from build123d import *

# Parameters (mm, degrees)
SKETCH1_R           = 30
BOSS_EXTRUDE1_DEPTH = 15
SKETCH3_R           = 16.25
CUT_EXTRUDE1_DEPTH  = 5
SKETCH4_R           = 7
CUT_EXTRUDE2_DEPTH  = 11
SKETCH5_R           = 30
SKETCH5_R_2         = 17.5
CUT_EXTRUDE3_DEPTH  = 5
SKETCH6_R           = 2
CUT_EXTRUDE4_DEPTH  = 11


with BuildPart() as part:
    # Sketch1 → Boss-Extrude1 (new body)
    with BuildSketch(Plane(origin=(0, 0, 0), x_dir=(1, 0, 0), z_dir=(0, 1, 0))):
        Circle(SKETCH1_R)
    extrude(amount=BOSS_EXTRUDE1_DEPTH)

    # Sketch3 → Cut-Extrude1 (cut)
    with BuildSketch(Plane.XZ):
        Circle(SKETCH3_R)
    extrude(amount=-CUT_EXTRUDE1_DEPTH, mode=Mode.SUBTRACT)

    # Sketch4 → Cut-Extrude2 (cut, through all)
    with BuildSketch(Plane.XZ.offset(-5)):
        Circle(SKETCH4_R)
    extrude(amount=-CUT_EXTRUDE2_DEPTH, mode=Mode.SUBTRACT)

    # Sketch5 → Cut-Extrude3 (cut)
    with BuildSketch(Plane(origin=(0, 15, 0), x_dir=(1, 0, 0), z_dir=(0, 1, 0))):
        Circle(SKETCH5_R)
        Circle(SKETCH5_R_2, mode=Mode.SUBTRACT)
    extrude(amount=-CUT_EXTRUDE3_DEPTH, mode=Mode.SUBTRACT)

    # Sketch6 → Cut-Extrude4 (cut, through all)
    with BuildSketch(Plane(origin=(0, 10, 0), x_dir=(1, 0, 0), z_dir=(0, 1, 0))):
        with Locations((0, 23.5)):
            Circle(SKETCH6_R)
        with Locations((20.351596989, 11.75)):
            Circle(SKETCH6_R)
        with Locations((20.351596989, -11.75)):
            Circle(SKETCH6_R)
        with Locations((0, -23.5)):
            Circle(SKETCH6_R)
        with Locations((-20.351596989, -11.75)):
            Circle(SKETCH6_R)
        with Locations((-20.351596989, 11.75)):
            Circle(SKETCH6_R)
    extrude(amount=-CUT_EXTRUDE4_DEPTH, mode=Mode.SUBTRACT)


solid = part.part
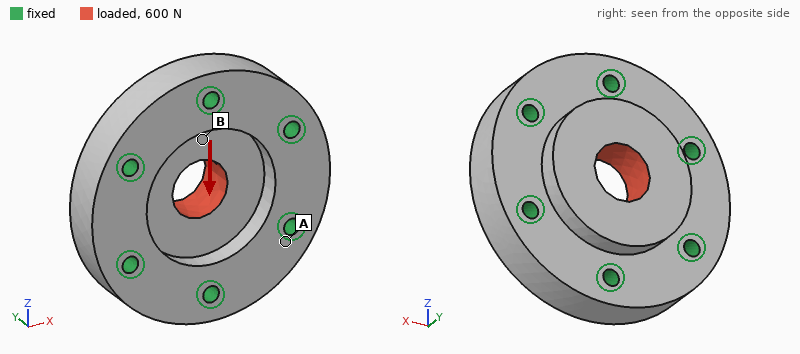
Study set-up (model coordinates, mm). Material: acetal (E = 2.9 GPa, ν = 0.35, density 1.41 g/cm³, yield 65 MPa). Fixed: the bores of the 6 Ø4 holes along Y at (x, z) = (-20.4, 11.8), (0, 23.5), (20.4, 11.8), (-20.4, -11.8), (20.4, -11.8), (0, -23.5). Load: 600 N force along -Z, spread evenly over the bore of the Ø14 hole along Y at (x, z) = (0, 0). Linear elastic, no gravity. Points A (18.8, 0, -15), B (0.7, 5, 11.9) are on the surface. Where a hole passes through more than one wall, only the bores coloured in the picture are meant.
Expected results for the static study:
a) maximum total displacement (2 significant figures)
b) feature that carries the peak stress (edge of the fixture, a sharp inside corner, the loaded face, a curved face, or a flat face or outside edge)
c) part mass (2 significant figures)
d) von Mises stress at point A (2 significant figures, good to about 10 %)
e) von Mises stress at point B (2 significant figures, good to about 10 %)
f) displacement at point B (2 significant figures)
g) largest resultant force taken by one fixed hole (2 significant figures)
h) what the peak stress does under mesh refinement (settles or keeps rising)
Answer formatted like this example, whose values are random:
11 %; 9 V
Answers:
13 µm; edge of the fixture; 38 g; 0.35 MPa; 1.7 MPa; 6.1 µm; 150 N; keeps rising
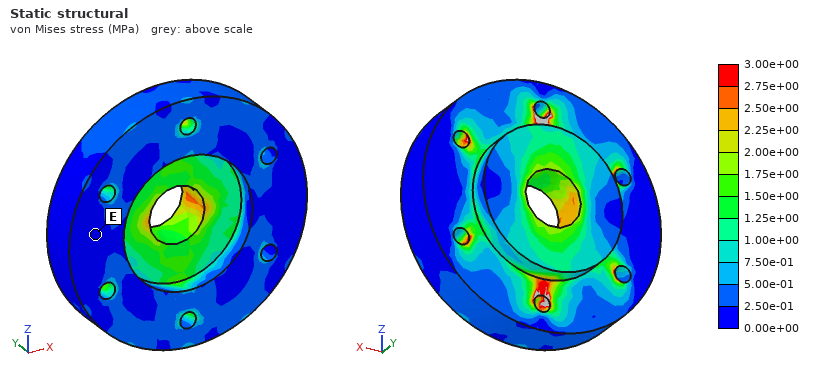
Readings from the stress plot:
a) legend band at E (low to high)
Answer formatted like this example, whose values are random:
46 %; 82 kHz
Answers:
0.00e+00 to 2.50e-01 MPa
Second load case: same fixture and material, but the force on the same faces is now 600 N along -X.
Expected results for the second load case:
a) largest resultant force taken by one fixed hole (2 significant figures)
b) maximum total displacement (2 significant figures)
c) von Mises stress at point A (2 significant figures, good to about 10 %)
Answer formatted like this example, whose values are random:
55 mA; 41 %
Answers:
130 N; 13 µm; 0.33 MPa
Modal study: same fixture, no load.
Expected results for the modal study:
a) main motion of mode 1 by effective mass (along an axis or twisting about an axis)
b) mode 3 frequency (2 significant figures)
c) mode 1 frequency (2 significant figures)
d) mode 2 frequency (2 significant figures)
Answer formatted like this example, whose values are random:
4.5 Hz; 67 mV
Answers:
along Y; 12 kHz; 9100 Hz; 12 kHz
